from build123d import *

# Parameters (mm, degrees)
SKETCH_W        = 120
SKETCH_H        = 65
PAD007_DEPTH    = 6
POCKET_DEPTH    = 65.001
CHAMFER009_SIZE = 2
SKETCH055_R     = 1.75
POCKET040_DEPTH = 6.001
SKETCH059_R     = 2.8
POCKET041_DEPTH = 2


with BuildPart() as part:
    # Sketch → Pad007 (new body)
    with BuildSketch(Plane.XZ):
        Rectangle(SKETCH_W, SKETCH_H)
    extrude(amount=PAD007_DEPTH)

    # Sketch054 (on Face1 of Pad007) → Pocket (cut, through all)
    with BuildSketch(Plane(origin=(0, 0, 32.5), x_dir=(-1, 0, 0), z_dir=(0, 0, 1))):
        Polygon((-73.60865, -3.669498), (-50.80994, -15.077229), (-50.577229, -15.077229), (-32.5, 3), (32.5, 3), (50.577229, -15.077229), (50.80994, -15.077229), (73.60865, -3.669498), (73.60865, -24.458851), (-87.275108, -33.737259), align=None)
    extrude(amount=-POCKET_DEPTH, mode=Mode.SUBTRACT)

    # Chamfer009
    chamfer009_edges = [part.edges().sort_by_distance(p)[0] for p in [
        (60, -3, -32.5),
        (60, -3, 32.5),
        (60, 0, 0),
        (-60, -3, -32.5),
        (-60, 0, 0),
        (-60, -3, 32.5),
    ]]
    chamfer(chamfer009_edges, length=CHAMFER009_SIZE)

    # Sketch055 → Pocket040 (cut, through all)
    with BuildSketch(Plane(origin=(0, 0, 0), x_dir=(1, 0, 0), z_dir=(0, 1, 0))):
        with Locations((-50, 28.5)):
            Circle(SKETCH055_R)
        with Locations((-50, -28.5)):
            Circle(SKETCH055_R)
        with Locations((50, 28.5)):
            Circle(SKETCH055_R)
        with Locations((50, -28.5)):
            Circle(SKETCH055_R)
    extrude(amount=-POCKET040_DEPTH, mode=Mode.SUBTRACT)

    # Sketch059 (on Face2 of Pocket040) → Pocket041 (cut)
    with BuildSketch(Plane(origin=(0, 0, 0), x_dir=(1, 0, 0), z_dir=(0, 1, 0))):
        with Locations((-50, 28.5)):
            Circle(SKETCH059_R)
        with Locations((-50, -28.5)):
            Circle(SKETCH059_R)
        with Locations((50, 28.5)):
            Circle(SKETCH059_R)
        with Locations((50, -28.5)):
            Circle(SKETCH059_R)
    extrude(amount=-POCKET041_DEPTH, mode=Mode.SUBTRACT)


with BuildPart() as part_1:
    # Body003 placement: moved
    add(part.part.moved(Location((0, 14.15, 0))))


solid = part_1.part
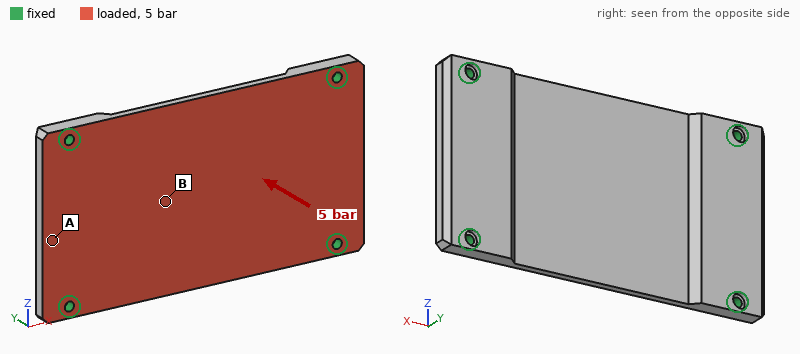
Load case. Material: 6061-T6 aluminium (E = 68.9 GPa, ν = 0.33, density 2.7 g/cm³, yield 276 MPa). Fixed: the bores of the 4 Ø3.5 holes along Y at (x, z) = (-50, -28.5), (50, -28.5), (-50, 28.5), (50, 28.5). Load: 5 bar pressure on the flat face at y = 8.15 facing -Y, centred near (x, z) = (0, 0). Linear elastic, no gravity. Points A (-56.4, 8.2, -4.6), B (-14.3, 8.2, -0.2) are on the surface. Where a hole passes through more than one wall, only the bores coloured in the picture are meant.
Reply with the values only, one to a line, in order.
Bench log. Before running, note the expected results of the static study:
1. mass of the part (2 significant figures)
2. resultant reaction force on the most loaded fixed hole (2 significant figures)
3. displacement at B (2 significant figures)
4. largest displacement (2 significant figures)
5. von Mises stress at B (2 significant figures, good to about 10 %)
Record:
89 g
1.5 kN
0.40 mm
0.48 mm
63 MPa
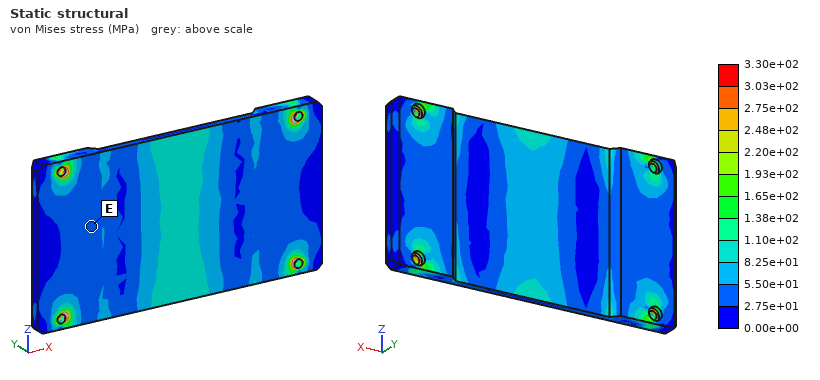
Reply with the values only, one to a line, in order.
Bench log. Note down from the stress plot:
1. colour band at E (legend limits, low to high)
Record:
2.75e+01 to 5.50e+01 MPa
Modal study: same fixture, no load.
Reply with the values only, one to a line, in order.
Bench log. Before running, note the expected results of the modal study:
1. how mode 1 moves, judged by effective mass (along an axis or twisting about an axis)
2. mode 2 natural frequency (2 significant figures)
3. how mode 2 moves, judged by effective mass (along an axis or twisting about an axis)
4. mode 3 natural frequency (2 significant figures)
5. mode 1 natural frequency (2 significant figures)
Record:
along Y
3200 Hz
twisting about X
4400 Hz
2100 Hz
